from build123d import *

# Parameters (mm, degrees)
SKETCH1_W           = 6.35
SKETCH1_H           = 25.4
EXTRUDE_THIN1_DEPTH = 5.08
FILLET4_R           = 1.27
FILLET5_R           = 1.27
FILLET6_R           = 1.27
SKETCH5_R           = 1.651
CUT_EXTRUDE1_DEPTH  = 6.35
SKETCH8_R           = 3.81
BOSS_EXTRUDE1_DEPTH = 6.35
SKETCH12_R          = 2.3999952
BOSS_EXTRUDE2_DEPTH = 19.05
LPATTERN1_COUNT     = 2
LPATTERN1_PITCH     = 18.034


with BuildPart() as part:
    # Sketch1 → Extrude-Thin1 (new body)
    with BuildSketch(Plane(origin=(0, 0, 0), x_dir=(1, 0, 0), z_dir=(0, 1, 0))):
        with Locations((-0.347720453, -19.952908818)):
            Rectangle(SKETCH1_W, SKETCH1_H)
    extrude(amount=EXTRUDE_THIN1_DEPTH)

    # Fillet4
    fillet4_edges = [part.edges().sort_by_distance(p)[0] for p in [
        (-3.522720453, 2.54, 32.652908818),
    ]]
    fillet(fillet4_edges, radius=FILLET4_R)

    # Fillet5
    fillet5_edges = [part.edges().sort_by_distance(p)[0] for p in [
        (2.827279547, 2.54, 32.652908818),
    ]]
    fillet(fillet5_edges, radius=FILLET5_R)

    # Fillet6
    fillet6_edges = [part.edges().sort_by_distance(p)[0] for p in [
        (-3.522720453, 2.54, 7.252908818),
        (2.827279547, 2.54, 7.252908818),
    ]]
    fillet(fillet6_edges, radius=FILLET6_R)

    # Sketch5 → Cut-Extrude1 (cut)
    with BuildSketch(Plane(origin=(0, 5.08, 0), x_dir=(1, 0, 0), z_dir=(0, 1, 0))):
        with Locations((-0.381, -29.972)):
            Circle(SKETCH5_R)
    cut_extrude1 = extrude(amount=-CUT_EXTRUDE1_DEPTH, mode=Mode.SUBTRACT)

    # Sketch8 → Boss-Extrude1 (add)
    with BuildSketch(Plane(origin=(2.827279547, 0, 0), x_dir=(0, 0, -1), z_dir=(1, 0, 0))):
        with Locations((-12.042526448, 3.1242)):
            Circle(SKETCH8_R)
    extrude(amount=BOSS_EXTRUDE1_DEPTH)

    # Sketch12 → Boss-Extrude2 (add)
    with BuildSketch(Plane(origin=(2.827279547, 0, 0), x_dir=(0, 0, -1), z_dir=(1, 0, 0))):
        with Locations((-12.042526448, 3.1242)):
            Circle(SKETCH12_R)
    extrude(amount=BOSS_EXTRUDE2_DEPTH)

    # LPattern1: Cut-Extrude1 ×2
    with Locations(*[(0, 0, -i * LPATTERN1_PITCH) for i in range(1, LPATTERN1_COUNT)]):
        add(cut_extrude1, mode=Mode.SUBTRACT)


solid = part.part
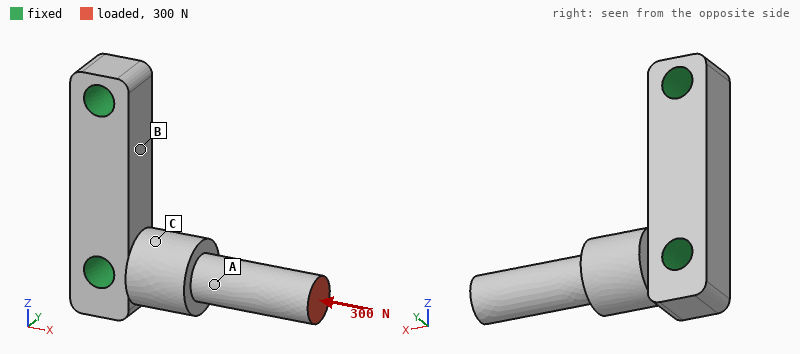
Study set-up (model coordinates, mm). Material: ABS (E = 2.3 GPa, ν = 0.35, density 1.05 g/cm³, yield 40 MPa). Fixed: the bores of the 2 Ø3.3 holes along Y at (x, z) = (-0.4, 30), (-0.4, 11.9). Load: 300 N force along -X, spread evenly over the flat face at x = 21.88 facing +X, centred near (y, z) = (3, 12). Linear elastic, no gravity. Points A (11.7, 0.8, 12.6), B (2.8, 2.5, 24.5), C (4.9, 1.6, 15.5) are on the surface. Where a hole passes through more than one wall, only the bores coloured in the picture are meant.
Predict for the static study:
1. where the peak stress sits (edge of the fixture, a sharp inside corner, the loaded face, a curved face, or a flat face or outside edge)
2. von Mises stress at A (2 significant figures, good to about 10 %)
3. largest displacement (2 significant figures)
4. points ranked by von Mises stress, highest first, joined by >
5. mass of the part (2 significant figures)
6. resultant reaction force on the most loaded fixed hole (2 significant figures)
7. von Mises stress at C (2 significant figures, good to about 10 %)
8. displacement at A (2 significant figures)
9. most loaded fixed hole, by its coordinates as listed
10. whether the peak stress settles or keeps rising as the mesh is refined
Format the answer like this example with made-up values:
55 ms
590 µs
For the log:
edge of the fixture
16 MPa
0.15 mm
A > C > B
1.3 g
290 N
6.1 MPa
0.053 mm
(-0.4, 11.9)
keeps rising
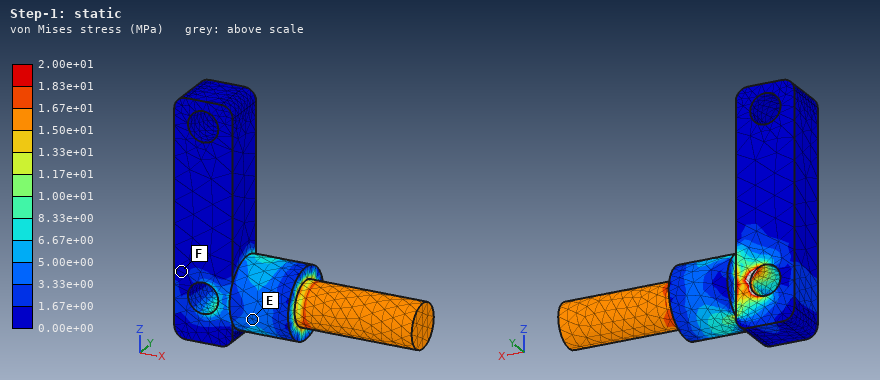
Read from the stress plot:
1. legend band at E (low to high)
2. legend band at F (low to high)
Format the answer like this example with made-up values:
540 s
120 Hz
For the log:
3.33e+00 to 5.00e+00 MPa
0.00e+00 to 1.67e+00 MPa
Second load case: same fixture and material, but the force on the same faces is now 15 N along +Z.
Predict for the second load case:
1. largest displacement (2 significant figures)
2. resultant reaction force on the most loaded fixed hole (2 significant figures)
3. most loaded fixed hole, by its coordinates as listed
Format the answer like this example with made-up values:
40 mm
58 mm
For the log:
0.34 mm
11 N
(-0.4, 11.9)
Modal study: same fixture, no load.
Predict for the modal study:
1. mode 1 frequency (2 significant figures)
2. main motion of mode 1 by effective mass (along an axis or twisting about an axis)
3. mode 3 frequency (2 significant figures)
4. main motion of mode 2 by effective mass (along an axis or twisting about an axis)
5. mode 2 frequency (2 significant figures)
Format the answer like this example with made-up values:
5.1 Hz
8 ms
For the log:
3400 Hz
along Y
12 kHz
along Z
3700 Hz
